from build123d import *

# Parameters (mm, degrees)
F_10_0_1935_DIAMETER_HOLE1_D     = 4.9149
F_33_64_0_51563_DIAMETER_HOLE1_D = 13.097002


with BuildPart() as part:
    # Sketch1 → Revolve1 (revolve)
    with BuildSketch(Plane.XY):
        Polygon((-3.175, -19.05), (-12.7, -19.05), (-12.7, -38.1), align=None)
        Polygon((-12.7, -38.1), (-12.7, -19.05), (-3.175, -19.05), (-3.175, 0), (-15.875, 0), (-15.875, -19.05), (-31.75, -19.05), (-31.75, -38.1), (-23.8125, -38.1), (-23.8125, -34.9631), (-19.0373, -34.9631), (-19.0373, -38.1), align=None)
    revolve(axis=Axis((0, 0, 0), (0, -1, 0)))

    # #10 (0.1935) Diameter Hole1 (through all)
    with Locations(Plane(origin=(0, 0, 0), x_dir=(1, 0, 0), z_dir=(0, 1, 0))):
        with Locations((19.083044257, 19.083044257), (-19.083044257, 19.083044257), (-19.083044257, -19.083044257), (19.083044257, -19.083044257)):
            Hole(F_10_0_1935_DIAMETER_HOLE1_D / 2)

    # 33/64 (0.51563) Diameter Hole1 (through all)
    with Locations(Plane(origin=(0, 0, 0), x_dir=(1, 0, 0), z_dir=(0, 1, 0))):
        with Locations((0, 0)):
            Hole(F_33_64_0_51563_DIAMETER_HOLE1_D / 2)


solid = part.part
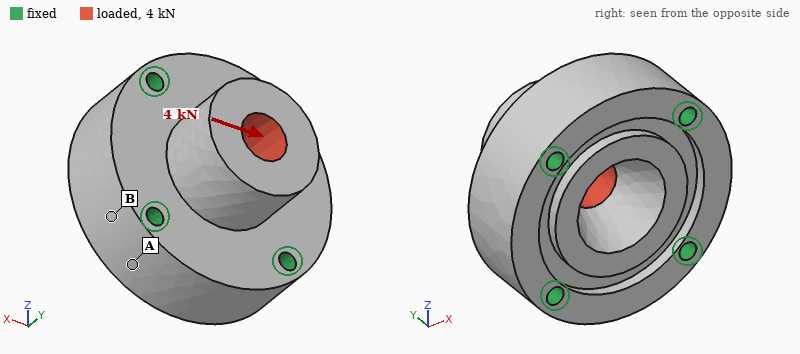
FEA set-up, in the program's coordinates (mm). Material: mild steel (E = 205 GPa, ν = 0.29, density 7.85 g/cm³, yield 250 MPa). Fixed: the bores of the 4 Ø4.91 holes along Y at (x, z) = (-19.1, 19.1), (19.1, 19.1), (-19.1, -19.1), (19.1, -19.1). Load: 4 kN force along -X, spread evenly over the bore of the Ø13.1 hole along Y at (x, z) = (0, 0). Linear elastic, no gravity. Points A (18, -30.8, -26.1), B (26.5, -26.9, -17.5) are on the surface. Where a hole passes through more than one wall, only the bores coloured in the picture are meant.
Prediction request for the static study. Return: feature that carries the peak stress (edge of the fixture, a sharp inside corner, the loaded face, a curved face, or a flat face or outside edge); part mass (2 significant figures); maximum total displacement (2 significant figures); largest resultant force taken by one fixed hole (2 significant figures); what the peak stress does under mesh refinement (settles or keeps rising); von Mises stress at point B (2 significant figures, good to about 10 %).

edge of the fixture
510 g
2.7 µm
1.3 kN
keeps rising
3.3 MPa
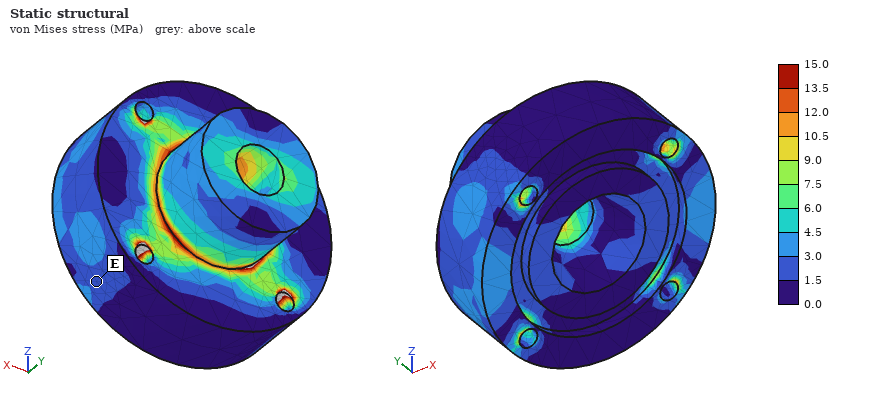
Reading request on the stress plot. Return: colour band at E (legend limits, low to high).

1.5 to 3.0 MPa
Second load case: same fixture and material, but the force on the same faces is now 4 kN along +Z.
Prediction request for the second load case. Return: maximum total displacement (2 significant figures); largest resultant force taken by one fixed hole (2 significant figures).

2.6 µm
1.3 kN
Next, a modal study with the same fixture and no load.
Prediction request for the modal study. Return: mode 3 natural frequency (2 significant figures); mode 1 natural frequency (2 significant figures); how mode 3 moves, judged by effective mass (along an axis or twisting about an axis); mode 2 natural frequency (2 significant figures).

22 kHz
19 kHz
along Y
19 kHz
